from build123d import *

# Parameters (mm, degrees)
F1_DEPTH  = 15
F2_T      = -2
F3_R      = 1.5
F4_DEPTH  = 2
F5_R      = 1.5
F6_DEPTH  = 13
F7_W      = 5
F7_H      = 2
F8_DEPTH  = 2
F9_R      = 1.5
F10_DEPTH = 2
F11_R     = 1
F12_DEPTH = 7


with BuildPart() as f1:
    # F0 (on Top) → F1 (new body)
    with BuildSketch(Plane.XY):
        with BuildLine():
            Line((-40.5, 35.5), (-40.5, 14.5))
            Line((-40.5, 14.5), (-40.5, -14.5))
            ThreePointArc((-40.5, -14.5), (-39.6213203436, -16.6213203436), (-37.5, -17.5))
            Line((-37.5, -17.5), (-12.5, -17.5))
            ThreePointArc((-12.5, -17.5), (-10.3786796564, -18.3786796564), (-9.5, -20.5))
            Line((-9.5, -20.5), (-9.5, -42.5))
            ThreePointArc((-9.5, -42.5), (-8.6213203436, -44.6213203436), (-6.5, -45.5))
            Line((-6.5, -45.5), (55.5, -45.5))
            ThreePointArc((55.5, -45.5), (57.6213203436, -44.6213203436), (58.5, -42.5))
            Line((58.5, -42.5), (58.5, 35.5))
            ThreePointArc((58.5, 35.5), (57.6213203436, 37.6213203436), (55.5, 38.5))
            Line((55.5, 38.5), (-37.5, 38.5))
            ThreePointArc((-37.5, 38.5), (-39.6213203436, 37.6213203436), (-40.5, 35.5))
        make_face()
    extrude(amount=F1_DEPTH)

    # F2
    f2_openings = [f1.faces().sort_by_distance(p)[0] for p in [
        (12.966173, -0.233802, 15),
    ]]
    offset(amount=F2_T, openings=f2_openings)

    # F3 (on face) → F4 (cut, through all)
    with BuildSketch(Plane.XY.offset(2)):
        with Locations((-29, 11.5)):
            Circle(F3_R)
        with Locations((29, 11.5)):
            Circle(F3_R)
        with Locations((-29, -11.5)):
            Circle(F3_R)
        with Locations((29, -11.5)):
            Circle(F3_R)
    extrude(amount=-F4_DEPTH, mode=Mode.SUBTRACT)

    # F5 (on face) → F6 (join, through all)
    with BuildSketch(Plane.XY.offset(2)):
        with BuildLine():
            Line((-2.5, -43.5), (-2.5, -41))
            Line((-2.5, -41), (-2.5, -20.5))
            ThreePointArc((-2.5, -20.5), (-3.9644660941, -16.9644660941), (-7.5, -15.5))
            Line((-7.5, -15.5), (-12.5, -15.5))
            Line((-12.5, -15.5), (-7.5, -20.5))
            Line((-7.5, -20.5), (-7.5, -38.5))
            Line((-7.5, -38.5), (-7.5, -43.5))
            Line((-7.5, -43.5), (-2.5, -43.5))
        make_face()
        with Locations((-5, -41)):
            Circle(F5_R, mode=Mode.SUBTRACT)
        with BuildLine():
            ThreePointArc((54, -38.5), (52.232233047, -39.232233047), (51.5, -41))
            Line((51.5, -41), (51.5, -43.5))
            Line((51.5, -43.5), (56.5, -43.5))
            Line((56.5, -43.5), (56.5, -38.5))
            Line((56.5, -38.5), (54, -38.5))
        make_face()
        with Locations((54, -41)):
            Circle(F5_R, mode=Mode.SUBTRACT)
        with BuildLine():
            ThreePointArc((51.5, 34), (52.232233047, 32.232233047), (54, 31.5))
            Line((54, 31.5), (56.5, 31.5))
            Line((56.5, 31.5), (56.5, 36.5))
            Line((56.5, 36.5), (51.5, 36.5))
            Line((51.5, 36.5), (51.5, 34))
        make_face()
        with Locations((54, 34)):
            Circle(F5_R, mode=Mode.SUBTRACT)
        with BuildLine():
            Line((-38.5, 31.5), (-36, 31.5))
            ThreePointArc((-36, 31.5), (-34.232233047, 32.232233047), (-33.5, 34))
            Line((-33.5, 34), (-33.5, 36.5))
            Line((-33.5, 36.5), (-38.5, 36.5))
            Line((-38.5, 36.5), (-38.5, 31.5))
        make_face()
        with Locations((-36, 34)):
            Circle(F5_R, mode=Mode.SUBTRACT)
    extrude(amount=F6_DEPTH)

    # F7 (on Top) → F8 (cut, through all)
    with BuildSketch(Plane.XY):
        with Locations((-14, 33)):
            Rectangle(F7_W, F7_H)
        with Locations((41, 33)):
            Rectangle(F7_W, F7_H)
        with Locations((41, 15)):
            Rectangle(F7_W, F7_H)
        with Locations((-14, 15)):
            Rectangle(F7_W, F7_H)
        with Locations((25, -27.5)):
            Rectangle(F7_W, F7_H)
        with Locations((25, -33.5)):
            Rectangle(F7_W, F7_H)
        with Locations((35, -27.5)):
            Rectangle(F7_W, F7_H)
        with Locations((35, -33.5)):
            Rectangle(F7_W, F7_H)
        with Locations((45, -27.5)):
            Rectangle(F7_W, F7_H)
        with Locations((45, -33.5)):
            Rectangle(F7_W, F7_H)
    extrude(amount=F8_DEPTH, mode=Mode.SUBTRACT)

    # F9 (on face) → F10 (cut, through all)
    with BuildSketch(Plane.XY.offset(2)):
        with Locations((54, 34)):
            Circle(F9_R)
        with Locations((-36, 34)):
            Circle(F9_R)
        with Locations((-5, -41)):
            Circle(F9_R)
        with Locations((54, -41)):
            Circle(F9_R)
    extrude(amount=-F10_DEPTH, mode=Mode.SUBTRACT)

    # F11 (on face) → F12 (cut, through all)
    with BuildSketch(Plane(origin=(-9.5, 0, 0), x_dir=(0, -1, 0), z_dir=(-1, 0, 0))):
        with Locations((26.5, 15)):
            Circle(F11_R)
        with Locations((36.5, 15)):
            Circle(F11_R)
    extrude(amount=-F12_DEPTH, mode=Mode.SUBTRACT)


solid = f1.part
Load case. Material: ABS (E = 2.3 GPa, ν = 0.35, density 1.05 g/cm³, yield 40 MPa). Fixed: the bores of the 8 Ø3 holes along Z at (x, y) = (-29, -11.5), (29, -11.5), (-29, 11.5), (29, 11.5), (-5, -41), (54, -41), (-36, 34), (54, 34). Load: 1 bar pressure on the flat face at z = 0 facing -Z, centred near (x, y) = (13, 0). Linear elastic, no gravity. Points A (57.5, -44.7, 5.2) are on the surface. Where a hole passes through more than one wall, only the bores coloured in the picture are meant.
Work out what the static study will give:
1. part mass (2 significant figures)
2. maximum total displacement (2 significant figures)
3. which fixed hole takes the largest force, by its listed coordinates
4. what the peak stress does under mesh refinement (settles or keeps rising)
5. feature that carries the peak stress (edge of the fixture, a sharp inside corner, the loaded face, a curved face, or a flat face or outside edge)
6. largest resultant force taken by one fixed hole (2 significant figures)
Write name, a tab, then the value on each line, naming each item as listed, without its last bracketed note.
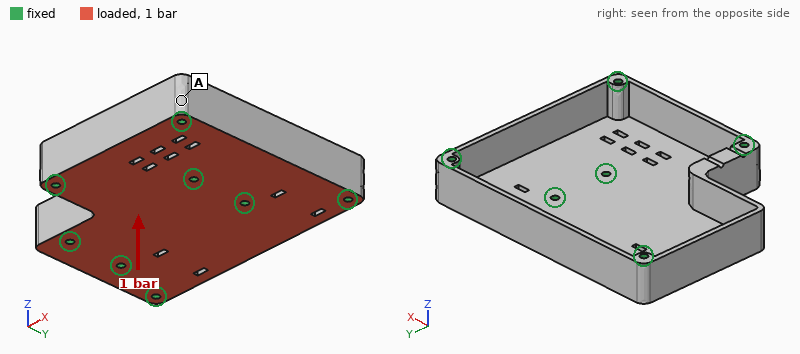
part mass	27 g
maximum total displacement	1.1 mm
which fixed hole takes the largest force, by its listed coordinates	(-5, -41)
what the peak stress does under mesh refinement	keeps rising
feature that carries the peak stress	edge of the fixture
largest resultant force taken by one fixed hole	160 N
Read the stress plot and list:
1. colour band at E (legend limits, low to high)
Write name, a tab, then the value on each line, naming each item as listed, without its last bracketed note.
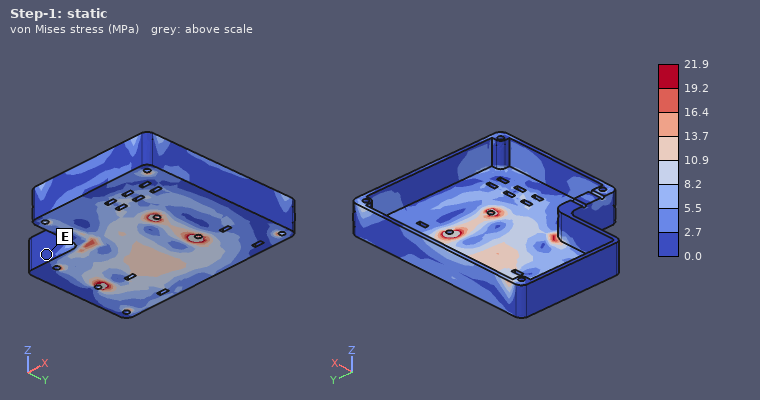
colour band at E	0.0 to 2.7 MPa
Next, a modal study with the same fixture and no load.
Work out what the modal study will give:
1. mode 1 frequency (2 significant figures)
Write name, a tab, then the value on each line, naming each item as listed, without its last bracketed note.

mode 1 frequency	1200 Hz
